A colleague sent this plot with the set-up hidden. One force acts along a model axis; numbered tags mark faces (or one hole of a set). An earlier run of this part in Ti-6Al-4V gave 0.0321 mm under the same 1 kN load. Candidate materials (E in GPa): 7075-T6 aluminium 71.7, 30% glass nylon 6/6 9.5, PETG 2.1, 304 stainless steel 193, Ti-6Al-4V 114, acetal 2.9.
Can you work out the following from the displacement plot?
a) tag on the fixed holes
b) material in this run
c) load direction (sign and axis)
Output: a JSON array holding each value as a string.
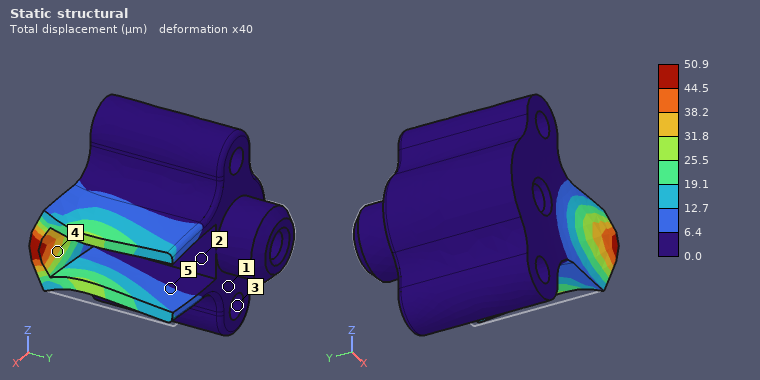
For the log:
["3", "7075-T6 aluminium", "-Y"]
